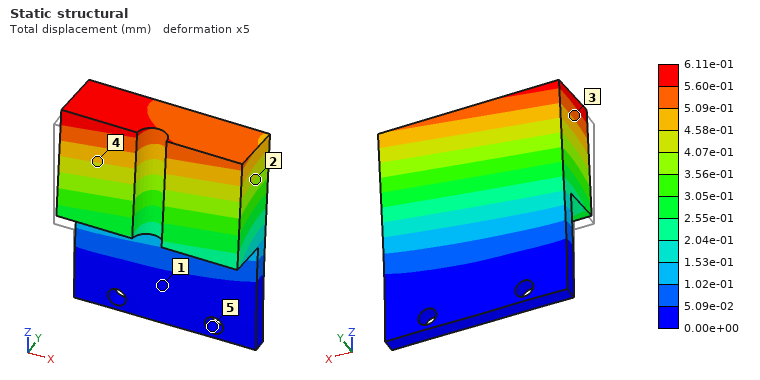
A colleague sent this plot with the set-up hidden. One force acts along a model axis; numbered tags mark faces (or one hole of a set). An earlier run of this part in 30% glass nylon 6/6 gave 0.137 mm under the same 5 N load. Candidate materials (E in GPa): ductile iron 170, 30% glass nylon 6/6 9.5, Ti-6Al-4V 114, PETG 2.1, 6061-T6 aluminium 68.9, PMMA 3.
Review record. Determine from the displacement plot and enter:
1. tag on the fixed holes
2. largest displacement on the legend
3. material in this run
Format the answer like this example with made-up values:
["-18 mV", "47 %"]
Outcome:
["5", "6.11e-01 mm", "PETG"]
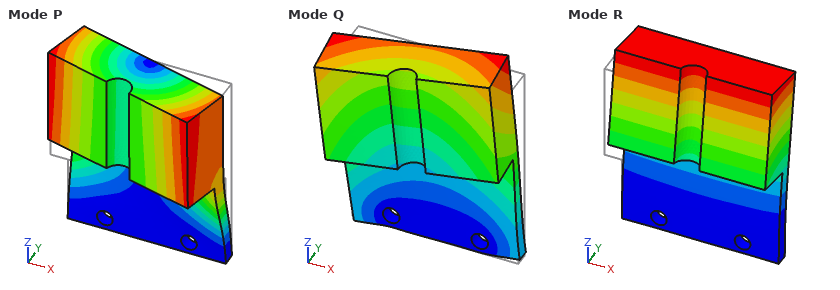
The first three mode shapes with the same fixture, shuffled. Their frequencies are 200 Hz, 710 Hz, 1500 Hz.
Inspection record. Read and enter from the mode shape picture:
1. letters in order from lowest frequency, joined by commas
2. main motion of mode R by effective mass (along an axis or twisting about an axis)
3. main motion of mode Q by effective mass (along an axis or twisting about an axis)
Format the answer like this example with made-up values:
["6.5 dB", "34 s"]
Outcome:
["R, P, Q", "along Y", "along X"]
